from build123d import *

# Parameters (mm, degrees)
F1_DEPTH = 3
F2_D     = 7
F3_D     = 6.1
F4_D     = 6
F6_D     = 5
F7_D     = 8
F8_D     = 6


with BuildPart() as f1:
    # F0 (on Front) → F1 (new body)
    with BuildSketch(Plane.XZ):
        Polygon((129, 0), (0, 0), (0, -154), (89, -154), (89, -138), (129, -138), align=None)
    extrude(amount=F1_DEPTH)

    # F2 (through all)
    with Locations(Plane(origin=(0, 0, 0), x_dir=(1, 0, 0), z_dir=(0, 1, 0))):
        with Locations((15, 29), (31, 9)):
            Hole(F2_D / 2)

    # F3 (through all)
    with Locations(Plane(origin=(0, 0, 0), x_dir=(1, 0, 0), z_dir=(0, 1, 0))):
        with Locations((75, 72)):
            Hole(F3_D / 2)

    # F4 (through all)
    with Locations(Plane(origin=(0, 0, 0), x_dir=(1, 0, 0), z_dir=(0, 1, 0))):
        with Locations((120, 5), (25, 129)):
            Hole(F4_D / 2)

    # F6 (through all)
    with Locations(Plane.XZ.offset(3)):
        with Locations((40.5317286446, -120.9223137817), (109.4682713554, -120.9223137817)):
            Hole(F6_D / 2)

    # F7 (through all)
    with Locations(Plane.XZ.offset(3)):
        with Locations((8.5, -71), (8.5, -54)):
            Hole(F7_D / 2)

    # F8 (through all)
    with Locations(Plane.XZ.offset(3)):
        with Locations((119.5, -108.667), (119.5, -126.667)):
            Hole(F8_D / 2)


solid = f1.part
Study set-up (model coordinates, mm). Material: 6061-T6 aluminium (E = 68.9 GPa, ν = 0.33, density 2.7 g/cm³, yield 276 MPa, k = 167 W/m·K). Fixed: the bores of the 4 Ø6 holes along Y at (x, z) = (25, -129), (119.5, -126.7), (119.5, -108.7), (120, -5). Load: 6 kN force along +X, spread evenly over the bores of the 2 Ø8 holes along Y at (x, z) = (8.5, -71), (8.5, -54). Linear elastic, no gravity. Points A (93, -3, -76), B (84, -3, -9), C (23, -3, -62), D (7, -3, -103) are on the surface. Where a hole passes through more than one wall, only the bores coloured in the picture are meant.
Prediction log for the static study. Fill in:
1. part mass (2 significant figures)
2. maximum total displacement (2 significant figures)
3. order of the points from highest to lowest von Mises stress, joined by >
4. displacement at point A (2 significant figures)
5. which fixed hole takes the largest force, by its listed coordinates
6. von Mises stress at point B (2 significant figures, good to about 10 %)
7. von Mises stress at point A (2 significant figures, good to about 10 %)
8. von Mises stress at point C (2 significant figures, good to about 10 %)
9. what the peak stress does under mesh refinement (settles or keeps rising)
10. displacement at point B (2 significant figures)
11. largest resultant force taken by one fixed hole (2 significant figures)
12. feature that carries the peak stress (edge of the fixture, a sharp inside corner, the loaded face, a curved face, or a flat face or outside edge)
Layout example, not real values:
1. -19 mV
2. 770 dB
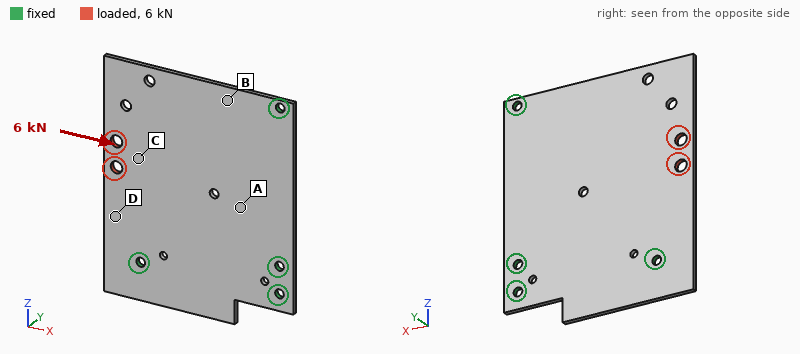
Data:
1. 150 g
2. 61 µm
3. C > B > A > D
4. 18 µm
5. (120, -5)
6. 23 MPa
7. 15 MPa
8. 46 MPa
9. keeps rising
10. 18 µm
11. 2.4 kN
12. edge of the fixture
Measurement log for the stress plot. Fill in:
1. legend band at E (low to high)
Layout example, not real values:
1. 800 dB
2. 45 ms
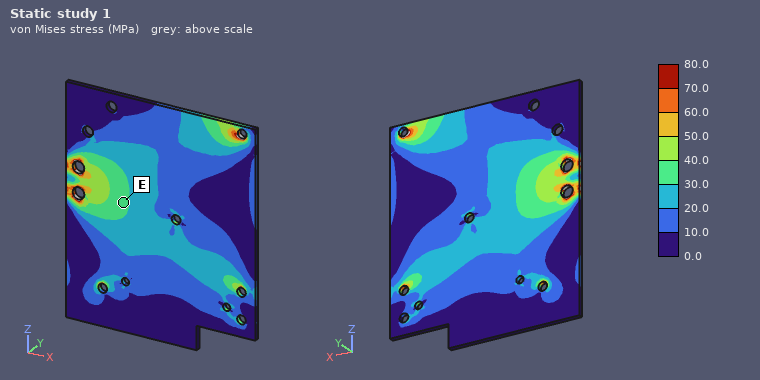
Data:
1. 30.0 to 40.0 MPa
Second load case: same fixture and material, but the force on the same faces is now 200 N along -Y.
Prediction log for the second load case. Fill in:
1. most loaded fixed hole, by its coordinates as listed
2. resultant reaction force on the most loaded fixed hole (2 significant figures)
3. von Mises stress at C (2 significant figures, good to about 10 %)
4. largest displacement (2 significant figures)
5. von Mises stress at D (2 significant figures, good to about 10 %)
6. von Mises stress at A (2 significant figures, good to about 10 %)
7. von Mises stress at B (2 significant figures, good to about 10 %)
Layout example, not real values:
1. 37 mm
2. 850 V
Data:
1. (25, -129)
2. 190 N
3. 41 MPa
4. 2.0 mm
5. 48 MPa
6. 19 MPa
7. 27 MPa
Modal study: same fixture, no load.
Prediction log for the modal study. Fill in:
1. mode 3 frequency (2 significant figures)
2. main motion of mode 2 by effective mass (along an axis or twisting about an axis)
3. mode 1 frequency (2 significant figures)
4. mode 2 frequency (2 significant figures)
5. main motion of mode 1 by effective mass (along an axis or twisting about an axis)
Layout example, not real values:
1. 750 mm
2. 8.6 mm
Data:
1. 1100 Hz
2. along Y
3. 300 Hz
4. 980 Hz
5. along Y
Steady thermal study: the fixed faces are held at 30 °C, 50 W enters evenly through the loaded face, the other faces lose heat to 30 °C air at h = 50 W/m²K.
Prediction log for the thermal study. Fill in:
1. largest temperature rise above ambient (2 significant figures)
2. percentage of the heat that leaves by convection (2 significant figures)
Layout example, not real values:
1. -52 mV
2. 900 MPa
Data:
1. 72 K
2. 57 %
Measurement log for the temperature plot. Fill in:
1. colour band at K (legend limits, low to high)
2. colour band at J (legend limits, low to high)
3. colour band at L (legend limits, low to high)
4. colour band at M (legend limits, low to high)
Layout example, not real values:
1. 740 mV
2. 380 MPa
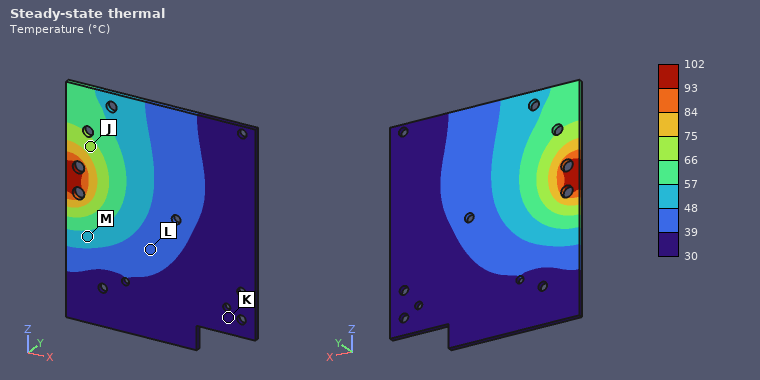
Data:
1. 30 to 39 °C
2. 66 to 75 °C
3. 39 to 48 °C
4. 48 to 57 °C
